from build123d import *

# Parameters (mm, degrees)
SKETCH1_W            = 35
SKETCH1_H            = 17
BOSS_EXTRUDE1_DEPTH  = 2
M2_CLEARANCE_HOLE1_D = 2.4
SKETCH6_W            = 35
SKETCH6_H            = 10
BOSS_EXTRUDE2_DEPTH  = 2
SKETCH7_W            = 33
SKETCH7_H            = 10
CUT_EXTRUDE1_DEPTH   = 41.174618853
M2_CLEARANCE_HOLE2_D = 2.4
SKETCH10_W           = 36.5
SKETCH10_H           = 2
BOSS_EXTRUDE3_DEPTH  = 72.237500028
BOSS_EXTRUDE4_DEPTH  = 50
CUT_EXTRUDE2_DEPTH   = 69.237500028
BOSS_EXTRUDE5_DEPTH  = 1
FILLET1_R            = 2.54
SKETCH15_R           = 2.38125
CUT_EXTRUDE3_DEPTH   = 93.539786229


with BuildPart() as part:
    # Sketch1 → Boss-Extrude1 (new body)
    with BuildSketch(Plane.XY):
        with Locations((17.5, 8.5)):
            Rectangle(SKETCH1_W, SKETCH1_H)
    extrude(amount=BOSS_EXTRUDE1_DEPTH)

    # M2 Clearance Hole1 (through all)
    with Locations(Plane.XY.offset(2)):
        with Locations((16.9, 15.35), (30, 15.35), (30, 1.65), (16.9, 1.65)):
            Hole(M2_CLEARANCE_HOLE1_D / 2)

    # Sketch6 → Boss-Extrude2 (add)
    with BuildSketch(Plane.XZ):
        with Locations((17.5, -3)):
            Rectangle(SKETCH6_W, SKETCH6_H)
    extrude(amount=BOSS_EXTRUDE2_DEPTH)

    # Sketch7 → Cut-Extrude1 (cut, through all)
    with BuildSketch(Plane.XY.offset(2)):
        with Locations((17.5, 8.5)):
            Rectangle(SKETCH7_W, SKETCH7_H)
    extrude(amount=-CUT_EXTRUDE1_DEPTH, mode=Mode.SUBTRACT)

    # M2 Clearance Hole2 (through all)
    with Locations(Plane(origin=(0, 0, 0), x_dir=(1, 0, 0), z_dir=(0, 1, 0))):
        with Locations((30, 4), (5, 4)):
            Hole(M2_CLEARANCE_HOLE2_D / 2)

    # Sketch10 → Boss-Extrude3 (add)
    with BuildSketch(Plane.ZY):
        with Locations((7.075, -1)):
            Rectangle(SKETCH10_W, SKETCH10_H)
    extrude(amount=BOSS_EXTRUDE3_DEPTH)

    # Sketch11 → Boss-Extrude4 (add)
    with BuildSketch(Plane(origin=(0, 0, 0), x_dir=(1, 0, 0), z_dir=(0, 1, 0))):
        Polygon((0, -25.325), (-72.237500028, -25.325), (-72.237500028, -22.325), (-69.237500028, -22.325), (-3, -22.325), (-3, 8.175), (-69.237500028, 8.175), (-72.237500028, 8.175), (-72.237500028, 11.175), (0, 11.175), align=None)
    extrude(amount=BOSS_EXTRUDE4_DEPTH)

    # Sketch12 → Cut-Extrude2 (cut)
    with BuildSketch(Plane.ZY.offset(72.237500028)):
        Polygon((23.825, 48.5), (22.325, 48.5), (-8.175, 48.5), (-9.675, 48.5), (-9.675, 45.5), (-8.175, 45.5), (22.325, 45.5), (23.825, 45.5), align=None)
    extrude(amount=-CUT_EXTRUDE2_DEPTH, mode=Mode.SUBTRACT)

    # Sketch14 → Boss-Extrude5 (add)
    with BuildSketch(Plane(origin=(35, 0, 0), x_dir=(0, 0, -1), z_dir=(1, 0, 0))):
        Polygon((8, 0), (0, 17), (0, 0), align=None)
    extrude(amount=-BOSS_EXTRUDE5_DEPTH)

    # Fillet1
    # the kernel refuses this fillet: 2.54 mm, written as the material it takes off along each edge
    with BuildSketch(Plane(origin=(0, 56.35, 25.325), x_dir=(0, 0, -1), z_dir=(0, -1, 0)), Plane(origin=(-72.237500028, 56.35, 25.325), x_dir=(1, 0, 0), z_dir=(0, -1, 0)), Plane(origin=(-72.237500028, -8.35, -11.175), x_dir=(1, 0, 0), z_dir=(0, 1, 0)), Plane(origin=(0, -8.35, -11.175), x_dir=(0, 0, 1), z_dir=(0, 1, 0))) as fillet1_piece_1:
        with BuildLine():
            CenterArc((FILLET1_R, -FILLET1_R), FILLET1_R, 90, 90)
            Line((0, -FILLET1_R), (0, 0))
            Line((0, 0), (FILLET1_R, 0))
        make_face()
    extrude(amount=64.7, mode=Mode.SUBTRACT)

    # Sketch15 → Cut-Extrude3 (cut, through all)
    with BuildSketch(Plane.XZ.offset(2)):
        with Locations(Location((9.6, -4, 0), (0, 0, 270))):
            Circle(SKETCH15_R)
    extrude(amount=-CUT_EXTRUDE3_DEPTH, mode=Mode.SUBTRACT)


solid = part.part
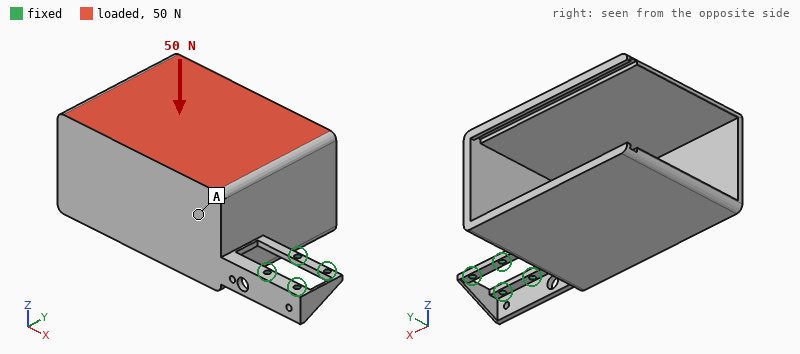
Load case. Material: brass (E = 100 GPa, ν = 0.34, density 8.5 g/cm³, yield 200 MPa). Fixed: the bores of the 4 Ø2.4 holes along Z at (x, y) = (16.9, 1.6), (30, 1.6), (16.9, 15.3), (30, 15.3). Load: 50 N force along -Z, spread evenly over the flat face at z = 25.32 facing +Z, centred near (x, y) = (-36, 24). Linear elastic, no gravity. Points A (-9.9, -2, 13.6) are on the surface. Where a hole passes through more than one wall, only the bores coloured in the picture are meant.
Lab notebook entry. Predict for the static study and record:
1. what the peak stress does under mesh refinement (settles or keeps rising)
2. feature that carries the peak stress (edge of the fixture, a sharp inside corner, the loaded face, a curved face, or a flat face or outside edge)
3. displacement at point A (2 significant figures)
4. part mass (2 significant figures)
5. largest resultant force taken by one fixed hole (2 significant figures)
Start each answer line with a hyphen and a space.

- keeps rising
- edge of the fixture
- 0.092 mm
- 270 g
- 200 N
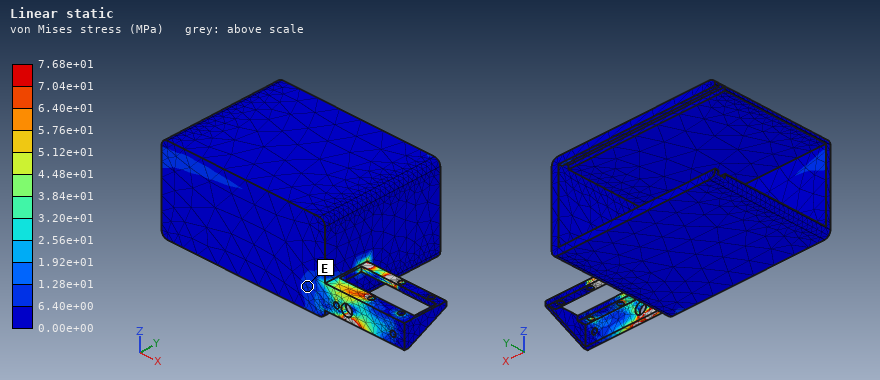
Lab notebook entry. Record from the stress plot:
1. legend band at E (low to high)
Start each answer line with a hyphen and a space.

- 6.40e+00 to 1.28e+01 MPa
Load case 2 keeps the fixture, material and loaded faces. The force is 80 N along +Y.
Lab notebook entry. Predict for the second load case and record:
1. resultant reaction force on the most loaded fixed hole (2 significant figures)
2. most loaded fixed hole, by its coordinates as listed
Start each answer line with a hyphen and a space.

- 240 N
- (16.9, 15.3)
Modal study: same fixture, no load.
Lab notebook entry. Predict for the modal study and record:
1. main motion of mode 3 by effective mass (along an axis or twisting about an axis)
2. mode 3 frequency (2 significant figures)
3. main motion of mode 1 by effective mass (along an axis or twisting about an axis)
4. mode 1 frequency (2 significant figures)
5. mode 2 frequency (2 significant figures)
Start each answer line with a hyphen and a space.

- along Y
- 360 Hz
- along Z
- 140 Hz
- 230 Hz
